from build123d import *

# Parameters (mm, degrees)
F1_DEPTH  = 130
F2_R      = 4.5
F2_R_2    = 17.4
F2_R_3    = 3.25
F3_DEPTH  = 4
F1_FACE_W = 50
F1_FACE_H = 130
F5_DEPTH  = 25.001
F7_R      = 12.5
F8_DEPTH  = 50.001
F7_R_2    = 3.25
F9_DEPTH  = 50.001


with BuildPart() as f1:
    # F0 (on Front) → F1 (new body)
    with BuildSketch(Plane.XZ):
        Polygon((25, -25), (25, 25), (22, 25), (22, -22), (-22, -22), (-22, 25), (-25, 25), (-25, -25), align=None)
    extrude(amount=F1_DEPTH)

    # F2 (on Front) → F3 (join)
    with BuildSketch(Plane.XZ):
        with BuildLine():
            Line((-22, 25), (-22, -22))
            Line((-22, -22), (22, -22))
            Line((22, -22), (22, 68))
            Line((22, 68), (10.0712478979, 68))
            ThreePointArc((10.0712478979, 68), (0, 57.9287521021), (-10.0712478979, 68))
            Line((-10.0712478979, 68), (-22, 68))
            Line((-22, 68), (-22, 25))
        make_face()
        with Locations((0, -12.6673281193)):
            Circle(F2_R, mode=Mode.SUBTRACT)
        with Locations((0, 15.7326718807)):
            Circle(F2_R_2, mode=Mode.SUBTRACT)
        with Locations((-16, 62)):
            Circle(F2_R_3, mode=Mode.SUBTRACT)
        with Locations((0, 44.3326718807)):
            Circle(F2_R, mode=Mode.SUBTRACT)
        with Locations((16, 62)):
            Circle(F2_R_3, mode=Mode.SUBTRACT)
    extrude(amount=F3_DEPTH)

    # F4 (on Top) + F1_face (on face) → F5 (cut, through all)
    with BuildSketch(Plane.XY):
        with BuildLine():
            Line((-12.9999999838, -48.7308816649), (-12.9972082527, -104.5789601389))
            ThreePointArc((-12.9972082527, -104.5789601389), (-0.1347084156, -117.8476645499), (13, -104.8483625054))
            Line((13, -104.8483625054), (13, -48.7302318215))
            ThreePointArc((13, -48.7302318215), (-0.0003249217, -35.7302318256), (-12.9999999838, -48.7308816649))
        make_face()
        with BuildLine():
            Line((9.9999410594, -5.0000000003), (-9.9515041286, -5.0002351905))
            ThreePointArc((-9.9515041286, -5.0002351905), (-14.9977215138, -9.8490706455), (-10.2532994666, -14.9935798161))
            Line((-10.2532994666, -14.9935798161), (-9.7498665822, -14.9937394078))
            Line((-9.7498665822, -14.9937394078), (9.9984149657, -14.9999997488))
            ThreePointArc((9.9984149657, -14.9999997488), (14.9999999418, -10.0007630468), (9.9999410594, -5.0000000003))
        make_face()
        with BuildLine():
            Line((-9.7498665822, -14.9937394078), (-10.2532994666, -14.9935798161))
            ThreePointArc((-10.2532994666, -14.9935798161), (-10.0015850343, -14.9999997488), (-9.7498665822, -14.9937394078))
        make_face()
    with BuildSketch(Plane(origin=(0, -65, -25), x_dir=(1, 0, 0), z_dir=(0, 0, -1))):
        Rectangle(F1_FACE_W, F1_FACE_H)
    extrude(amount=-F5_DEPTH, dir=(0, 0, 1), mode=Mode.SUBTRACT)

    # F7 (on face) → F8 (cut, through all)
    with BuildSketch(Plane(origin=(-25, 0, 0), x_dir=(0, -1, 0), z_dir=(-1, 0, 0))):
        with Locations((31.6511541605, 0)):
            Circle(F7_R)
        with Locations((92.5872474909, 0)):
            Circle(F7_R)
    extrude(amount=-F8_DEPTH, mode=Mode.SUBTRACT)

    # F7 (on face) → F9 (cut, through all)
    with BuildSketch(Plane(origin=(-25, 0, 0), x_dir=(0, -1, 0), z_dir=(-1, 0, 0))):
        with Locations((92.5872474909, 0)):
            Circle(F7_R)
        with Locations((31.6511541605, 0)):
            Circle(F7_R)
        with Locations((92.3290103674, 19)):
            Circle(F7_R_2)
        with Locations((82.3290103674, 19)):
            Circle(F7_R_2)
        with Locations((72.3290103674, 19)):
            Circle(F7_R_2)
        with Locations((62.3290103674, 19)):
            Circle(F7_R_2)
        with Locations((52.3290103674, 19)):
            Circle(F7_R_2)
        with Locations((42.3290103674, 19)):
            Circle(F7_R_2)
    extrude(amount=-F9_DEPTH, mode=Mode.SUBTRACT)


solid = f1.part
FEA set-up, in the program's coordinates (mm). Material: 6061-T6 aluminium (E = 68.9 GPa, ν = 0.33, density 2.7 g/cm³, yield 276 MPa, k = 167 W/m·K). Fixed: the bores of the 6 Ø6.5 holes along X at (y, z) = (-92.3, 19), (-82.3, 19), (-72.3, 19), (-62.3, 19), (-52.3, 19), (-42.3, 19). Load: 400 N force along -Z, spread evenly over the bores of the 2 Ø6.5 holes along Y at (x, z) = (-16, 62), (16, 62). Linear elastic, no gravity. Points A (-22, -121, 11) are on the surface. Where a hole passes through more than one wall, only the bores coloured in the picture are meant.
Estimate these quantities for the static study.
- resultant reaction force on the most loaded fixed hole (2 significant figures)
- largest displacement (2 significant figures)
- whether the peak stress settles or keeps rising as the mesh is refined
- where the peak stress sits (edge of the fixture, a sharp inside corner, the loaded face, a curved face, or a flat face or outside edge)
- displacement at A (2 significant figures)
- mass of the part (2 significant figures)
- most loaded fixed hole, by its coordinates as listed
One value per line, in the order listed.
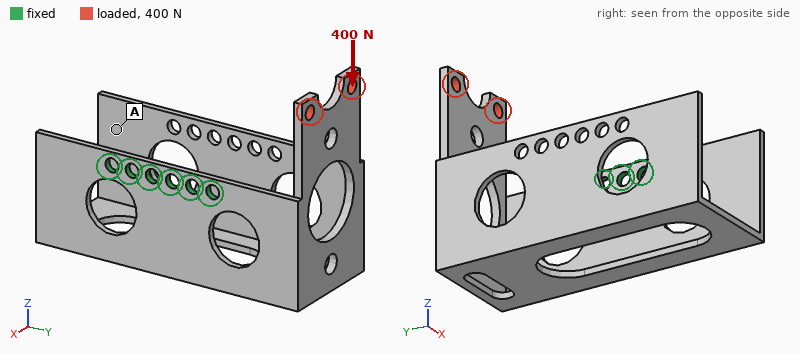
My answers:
630 N
1.9 mm
keeps rising
edge of the fixture
1.2 mm
140 g
(-42.3, 19)
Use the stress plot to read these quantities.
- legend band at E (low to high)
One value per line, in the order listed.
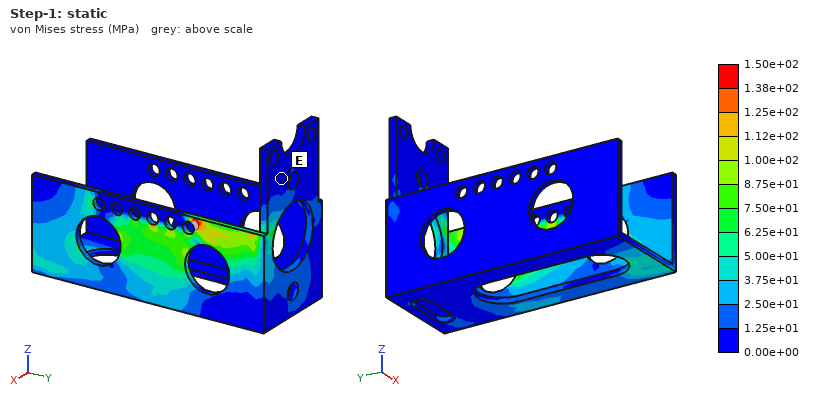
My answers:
0.00e+00 to 1.25e+01 MPa
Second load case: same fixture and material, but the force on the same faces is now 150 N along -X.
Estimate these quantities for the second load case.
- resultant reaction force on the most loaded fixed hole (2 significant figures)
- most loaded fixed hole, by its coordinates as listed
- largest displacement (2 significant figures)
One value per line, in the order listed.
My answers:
260 N
(-42.3, 19)
1.7 mm
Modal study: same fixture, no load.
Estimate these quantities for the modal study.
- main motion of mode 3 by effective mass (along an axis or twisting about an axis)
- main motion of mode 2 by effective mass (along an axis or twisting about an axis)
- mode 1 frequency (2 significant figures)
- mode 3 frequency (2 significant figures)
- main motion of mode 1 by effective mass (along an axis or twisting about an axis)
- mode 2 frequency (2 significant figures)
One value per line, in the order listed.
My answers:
along X
along Y
210 Hz
450 Hz
along Z
280 Hz
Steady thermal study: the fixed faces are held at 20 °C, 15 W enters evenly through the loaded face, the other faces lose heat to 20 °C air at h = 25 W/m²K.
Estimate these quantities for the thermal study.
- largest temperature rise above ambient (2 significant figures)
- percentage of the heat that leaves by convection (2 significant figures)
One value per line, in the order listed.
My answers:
54 K
63 %
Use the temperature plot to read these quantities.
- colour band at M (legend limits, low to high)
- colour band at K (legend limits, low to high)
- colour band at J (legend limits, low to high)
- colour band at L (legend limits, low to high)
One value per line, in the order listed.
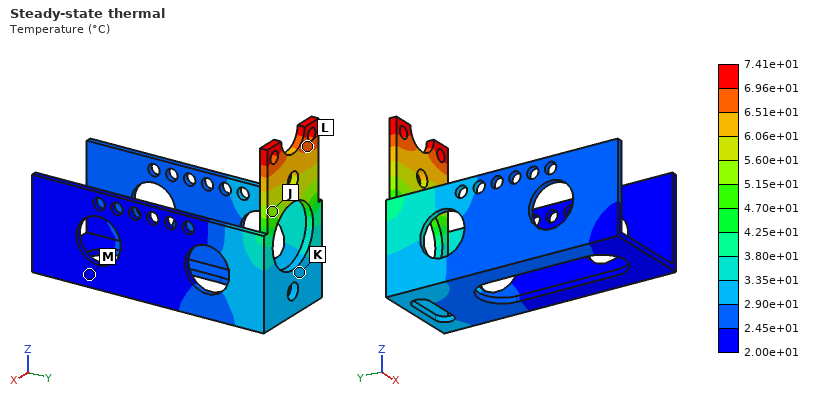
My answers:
2.00e+01 to 2.45e+01 °C
2.90e+01 to 3.35e+01 °C
5.15e+01 to 5.60e+01 °C
6.51e+01 to 6.96e+01 °C
